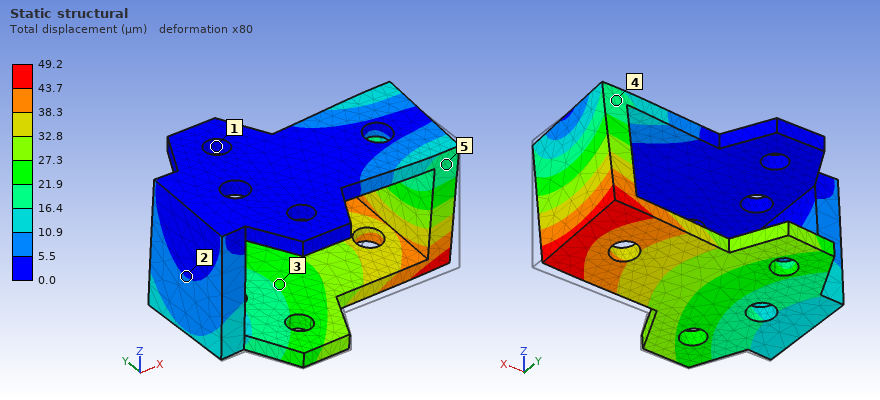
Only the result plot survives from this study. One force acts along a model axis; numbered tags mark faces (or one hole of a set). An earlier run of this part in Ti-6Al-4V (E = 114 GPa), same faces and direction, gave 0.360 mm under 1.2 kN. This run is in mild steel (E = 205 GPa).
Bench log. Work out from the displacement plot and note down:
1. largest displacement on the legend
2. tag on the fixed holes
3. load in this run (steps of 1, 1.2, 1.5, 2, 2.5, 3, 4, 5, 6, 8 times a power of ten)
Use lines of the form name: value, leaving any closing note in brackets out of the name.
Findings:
largest displacement on the legend: 49.2 µm
tag on the fixed holes: 1
load in this run: 300 N
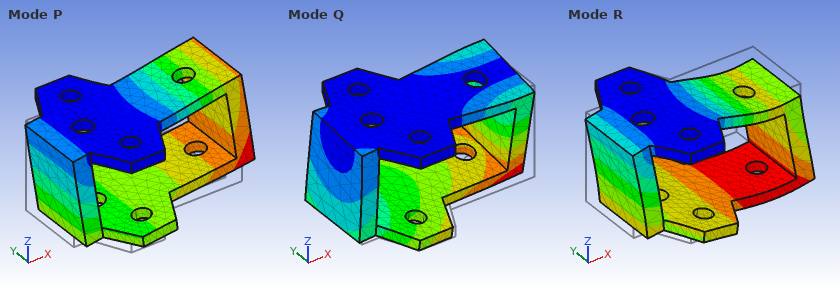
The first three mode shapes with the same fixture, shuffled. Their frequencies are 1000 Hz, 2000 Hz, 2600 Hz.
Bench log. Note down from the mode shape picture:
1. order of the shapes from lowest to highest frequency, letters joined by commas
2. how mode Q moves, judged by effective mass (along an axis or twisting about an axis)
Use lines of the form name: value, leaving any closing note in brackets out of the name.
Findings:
order of the shapes from lowest to highest frequency, letters joined by commas: P, Q, R
how mode Q moves, judged by effective mass: along Y
